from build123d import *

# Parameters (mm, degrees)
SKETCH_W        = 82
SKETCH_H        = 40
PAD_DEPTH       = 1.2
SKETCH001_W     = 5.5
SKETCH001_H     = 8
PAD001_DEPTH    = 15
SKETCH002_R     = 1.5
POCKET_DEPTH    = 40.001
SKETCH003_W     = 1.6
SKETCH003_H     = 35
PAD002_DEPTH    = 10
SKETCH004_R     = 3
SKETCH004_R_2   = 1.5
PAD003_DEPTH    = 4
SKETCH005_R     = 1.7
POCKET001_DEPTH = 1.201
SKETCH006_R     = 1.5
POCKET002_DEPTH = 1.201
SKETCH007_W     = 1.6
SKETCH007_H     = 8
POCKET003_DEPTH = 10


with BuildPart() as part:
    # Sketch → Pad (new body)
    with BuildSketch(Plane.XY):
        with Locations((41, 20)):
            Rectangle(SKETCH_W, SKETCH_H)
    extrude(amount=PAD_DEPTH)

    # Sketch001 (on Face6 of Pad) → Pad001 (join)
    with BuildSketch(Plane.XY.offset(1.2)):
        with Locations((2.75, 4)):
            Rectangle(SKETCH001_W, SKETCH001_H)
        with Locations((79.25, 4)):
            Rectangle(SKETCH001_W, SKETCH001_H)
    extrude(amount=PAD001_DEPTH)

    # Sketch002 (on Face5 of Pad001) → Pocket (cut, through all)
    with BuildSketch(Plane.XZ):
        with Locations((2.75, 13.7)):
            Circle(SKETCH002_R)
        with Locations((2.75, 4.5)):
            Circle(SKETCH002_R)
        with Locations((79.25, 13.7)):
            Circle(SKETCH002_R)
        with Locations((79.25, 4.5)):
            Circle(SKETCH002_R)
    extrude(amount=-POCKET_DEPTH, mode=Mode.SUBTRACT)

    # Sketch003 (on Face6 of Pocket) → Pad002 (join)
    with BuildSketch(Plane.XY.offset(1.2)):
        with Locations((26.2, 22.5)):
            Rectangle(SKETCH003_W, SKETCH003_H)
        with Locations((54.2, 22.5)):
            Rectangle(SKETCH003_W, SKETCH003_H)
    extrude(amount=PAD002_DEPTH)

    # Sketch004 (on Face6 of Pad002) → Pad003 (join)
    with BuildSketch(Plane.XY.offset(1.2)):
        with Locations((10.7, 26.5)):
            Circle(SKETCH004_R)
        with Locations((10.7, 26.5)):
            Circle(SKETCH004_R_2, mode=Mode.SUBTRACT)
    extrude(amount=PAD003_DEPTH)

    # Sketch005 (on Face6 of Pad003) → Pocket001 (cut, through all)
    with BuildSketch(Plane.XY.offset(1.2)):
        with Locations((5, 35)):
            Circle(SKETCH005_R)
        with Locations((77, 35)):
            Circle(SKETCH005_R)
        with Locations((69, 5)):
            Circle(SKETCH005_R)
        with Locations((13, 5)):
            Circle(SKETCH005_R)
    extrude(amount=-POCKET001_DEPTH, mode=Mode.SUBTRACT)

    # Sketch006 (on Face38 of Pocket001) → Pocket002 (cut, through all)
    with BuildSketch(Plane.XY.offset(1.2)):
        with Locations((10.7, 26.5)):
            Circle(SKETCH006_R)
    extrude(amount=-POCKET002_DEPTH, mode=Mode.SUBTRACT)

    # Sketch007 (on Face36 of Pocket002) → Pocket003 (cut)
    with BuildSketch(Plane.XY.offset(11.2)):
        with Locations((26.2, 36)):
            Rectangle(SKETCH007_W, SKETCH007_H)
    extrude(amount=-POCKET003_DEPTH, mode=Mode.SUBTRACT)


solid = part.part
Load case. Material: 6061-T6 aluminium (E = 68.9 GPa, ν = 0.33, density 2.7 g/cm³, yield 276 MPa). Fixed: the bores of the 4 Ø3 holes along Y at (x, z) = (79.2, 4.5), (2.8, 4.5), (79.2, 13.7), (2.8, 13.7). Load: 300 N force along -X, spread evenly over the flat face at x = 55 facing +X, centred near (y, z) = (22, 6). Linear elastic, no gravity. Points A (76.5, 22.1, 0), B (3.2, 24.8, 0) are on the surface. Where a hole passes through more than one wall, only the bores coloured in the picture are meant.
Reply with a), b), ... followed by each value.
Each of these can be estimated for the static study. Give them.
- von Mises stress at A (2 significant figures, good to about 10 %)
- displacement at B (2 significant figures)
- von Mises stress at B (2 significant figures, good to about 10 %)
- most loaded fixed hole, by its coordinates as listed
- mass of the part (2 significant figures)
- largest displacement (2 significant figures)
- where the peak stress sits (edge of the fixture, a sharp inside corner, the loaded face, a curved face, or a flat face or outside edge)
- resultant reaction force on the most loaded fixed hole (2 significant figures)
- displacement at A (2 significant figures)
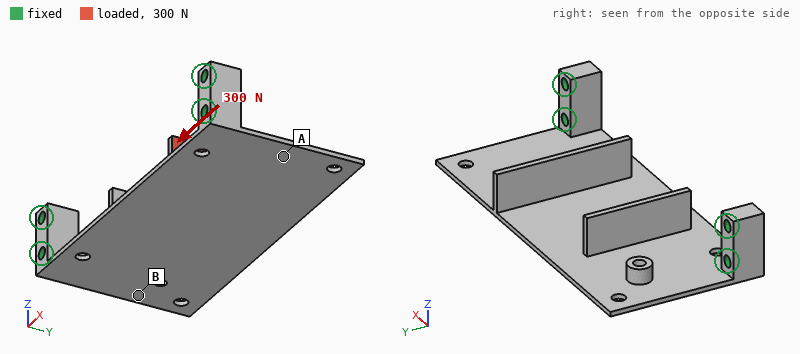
a) 30 MPa
b) 0.099 mm
c) 11 MPa
d) (79.2, 4.5)
e) 16 g
f) 0.54 mm
g) a flat face or outside edge
h) 190 N
i) 0.11 mm
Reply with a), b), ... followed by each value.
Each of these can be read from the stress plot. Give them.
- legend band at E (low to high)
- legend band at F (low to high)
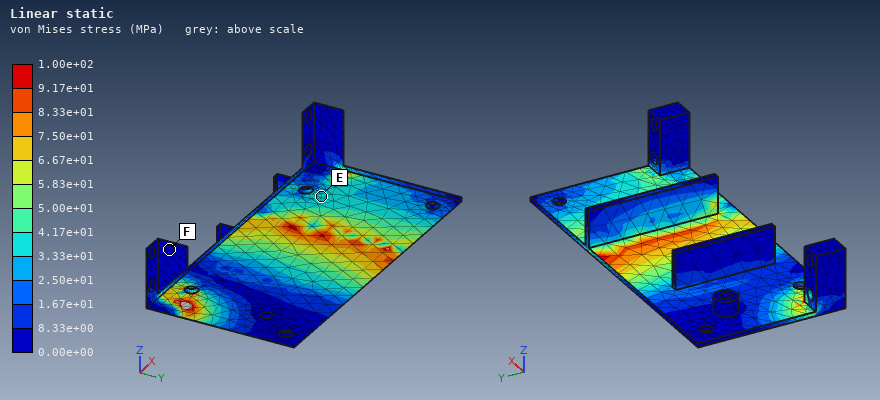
a) 3.33e+01 to 4.17e+01 MPa
b) 0.00e+00 to 8.33e+00 MPa
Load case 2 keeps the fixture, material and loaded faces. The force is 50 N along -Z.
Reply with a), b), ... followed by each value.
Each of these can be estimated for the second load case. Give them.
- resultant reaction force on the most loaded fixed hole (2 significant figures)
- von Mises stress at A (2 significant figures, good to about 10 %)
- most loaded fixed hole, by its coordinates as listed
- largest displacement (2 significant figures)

a) 37 N
b) 21 MPa
c) (79.2, 4.5)
d) 0.94 mm
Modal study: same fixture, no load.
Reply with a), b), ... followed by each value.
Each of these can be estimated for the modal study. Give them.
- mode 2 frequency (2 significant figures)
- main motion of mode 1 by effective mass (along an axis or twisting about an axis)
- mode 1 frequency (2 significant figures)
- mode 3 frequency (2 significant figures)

a) 1100 Hz
b) along Z
c) 480 Hz
d) 1200 Hz
